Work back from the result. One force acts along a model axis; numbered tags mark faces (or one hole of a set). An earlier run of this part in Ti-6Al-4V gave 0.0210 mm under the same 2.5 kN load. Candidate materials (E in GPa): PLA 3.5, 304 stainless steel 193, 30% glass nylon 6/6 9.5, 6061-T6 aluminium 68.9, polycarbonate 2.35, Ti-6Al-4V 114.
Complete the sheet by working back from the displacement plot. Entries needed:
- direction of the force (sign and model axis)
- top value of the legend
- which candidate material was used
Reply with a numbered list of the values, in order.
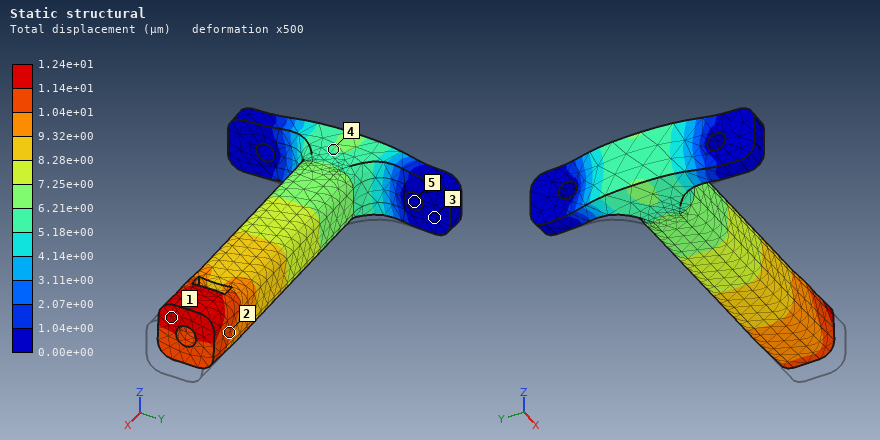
1. -X
2. 1.24e+01 µm
3. 304 stainless steel
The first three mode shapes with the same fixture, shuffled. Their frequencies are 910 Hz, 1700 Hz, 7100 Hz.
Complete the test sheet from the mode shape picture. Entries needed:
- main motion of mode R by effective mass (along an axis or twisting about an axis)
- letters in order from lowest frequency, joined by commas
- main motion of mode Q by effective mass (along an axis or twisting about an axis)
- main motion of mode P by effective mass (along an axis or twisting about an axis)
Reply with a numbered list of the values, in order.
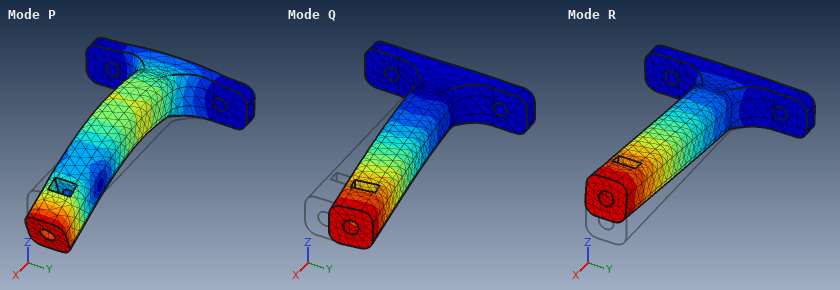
1. along Z
2. R, Q, P
3. along Y
4. along Z
